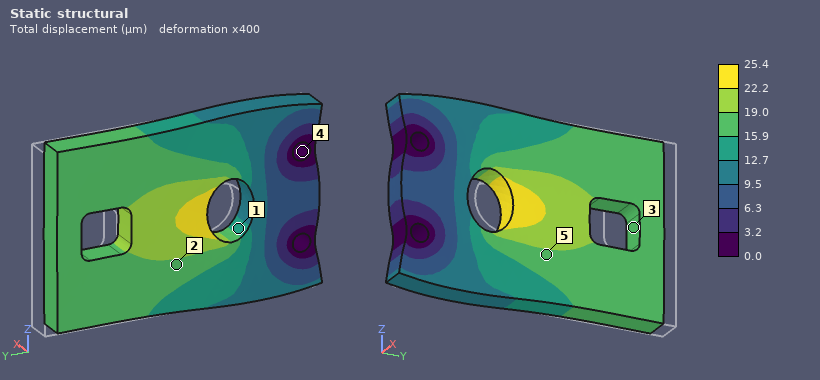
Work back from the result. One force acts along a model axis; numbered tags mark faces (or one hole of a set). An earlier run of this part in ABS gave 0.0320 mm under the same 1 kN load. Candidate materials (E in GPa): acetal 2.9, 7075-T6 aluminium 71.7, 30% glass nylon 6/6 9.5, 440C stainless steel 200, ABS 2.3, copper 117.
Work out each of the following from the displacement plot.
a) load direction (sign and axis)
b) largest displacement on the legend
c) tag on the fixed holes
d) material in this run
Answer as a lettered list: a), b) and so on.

a) -Y
b) 25.4 µm
c) 4
d) acetal
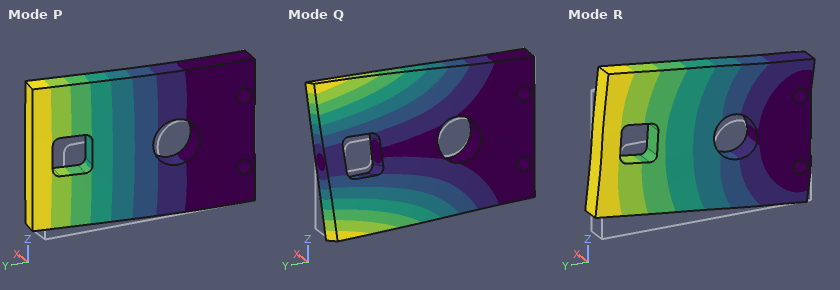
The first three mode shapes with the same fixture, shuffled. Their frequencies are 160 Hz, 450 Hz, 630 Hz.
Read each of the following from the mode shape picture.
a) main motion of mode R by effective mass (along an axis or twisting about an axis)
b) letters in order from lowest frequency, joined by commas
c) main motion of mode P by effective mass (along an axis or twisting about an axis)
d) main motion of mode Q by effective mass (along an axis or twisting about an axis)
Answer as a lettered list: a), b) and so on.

a) along Z
b) P, Q, R
c) along X
d) twisting about Y
